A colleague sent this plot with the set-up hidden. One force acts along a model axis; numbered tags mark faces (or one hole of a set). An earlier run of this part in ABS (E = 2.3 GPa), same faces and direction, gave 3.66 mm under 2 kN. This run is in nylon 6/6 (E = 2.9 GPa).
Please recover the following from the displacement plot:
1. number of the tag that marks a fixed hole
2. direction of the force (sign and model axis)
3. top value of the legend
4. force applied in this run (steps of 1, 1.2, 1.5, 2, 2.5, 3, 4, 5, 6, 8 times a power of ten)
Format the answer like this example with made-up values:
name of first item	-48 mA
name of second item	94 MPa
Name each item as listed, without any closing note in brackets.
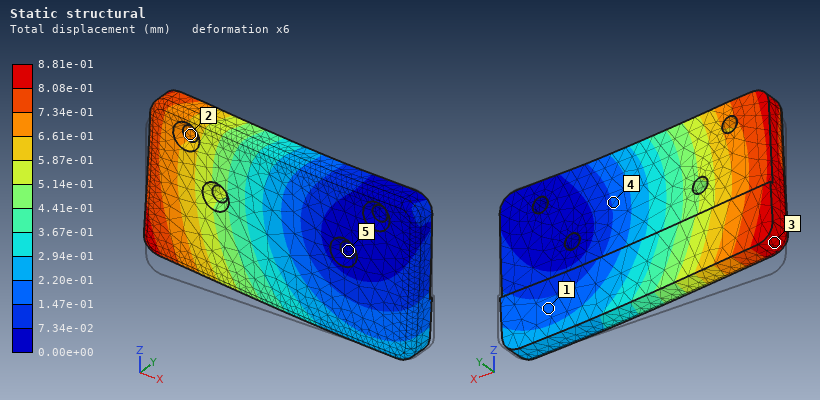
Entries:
number of the tag that marks a fixed hole	5
direction of the force	+Z
top value of the legend	8.81e-01 mm
force applied in this run	600 N
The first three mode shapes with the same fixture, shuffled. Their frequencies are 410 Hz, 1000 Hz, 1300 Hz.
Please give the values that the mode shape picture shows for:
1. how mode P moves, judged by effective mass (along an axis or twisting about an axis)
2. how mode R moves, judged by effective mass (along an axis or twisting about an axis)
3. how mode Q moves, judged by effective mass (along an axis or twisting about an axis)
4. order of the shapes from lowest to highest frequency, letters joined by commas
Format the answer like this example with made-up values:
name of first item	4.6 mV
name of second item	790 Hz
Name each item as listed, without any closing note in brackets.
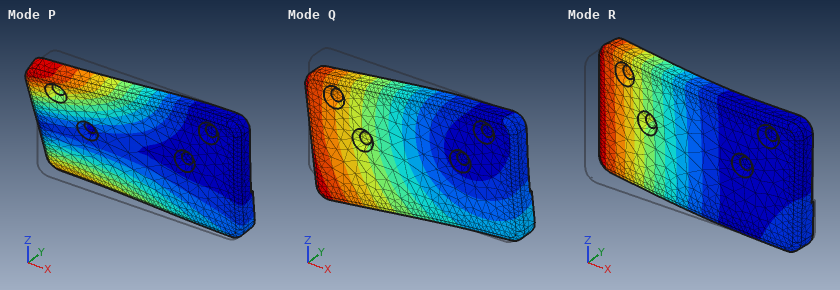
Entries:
how mode P moves, judged by effective mass	twisting about X
how mode R moves, judged by effective mass	along Y
how mode Q moves, judged by effective mass	along Z
order of the shapes from lowest to highest frequency, letters joined by commas	R, P, Q
